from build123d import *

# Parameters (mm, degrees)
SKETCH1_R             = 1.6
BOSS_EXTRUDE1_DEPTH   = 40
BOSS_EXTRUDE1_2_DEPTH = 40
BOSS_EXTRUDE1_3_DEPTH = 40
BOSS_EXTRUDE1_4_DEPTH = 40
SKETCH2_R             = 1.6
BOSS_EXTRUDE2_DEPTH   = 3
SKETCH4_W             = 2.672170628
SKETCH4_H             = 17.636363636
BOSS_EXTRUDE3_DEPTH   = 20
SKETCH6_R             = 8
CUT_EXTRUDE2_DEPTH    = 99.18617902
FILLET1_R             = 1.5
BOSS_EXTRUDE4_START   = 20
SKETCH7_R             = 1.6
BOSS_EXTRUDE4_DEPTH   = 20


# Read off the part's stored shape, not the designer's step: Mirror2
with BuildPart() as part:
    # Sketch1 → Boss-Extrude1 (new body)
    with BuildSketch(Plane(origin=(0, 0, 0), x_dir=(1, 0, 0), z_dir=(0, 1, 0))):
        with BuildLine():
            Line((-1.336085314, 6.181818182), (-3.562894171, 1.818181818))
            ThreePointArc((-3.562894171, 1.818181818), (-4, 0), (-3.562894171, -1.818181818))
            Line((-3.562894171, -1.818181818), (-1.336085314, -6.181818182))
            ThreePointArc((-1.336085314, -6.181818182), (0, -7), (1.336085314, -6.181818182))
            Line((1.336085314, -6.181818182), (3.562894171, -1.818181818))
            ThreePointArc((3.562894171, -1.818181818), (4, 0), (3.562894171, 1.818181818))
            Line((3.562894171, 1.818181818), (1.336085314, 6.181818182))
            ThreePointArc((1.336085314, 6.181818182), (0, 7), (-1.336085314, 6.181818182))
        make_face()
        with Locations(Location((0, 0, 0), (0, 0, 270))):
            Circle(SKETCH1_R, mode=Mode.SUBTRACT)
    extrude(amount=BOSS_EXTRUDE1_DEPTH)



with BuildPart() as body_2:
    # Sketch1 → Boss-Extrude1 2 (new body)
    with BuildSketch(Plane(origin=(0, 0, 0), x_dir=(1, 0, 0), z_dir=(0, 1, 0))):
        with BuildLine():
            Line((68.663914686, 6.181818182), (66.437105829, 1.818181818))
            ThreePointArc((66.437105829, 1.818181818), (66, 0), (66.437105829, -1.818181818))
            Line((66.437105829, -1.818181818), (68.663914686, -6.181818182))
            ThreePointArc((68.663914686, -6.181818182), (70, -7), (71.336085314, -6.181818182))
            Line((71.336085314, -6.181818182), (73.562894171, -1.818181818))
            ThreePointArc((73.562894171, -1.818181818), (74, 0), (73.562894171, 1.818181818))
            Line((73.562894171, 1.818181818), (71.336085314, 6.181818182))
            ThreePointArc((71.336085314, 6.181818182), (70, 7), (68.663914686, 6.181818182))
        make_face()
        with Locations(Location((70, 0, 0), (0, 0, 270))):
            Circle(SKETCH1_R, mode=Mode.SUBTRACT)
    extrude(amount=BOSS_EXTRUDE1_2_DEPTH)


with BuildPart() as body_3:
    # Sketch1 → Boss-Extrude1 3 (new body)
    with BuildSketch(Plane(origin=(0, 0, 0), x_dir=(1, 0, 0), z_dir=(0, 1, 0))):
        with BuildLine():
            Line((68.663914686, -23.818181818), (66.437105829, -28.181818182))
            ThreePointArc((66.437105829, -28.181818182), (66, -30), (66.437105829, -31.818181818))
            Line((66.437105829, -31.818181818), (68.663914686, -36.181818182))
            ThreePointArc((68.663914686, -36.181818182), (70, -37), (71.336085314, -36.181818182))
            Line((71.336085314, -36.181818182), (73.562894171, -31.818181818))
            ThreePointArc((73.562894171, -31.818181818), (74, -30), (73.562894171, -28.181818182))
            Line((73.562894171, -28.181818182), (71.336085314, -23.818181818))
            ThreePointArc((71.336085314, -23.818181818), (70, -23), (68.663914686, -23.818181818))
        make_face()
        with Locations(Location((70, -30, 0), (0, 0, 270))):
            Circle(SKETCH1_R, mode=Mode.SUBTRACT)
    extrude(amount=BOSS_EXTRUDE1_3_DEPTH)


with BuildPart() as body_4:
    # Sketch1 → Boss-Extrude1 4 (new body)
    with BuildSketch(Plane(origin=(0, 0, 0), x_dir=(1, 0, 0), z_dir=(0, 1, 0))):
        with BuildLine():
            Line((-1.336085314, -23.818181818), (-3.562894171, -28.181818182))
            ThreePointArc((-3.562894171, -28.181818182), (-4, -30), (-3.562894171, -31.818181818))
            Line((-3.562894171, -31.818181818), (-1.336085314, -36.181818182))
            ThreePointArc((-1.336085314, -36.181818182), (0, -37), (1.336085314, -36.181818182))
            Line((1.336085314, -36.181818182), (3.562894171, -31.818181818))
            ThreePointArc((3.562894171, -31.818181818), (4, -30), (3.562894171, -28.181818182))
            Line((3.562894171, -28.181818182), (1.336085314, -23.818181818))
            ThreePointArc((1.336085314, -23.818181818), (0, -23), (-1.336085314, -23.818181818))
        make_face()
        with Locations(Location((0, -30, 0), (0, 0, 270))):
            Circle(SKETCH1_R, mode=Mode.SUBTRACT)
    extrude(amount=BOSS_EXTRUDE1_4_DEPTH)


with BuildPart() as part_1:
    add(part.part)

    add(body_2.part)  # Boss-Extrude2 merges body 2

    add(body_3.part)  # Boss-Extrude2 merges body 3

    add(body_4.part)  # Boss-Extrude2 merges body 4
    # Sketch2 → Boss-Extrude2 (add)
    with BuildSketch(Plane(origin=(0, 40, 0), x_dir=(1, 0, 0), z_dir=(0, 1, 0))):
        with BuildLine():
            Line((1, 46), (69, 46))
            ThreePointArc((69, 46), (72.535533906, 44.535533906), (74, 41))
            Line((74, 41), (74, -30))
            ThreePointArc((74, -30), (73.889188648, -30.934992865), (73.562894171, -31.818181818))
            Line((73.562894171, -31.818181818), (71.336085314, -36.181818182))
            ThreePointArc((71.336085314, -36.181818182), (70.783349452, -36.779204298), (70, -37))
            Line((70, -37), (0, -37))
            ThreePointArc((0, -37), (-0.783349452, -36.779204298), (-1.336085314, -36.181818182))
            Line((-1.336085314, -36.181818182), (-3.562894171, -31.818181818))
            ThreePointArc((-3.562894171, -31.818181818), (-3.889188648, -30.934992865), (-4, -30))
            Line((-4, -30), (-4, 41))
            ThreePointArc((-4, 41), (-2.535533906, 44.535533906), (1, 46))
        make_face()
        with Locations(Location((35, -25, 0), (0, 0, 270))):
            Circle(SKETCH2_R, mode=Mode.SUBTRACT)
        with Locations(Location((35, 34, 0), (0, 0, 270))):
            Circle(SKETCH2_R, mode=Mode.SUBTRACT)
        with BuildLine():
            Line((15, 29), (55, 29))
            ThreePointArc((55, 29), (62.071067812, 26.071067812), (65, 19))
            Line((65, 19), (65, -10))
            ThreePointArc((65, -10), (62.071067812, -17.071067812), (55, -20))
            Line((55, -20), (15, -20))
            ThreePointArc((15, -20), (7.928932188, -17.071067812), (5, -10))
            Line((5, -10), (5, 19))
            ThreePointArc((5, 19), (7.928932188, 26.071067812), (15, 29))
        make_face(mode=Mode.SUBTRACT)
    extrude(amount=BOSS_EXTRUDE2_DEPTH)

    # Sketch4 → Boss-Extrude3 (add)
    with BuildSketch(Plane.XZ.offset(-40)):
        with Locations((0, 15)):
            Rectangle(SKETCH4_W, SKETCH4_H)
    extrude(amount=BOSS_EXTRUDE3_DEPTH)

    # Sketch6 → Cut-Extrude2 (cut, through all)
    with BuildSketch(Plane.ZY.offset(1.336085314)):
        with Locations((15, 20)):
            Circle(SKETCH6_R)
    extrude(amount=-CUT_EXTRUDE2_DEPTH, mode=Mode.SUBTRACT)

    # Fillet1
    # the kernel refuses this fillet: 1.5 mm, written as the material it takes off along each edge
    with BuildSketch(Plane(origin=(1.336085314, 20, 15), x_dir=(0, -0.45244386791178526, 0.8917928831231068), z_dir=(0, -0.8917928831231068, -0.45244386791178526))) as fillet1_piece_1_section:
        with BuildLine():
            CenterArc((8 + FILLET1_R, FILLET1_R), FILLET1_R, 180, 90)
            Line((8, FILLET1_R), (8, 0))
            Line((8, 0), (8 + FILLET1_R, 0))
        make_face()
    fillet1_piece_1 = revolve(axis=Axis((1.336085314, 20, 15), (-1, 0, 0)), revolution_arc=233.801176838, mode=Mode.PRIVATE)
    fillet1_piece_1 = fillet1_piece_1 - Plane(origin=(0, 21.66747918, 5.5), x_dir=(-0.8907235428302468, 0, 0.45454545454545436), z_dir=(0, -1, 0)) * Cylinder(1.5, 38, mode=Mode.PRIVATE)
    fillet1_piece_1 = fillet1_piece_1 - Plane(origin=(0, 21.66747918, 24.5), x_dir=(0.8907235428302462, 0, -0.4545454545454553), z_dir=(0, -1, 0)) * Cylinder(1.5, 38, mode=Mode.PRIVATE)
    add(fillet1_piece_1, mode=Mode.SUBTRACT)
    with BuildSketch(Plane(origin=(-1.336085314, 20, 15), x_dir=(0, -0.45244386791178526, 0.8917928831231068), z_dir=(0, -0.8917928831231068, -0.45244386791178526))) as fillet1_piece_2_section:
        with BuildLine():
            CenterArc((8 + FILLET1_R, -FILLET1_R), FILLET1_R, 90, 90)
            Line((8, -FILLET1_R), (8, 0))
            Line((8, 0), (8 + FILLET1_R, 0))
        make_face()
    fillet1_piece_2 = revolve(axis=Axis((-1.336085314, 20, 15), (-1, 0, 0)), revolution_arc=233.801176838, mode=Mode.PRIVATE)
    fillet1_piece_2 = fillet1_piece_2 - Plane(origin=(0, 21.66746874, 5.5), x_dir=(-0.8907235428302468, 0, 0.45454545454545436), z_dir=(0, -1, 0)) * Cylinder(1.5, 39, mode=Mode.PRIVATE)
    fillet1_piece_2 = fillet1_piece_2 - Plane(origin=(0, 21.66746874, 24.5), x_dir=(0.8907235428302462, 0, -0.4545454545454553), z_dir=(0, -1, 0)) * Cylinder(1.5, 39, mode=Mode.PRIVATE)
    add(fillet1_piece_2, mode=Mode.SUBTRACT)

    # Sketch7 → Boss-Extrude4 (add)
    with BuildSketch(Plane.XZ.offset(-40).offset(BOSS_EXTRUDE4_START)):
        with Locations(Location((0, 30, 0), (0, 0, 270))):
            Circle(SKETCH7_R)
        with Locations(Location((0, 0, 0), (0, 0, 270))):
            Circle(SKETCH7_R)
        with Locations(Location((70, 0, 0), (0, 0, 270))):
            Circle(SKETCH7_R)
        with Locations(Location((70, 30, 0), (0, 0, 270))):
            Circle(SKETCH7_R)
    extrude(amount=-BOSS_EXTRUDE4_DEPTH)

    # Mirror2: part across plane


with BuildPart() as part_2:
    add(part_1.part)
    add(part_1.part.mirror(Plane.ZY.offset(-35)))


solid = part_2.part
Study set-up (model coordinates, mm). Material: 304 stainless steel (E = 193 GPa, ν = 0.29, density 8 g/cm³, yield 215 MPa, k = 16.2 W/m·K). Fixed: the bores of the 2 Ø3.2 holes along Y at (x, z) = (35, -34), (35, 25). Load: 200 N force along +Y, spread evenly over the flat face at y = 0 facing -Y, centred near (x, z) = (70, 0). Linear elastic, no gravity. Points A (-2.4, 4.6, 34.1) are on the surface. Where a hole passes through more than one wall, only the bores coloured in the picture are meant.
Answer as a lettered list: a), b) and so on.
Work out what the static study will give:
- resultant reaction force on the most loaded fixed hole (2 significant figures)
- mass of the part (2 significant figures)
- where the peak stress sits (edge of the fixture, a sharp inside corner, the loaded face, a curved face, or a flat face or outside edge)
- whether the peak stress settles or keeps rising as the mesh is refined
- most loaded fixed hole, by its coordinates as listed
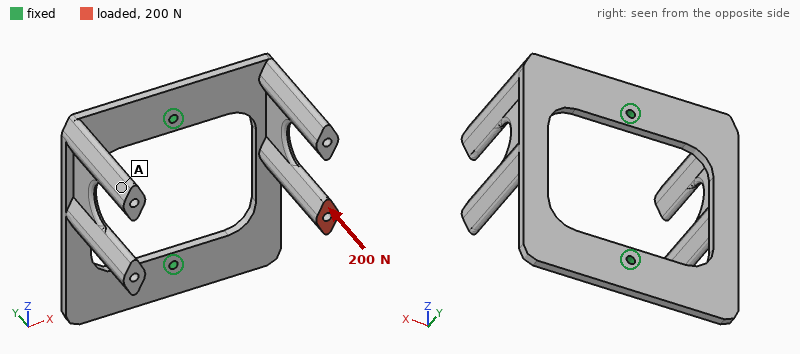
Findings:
a) 110 N
b) 180 g
c) edge of the fixture
d) keeps rising
e) (35, 25)
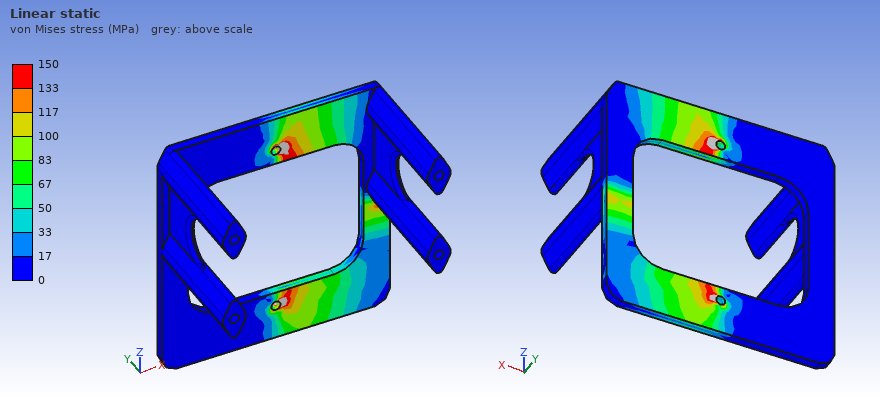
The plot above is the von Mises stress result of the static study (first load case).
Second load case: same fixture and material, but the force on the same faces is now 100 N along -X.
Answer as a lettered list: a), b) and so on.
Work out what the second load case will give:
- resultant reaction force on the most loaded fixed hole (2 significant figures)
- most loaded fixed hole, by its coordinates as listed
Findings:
a) 67 N
b) (35, 25)
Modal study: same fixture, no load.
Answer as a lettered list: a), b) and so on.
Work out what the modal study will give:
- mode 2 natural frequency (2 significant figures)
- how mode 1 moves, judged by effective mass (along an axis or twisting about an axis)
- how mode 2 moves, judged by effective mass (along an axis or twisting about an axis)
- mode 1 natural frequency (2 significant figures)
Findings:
a) 430 Hz
b) along X
c) along Y
d) 410 Hz
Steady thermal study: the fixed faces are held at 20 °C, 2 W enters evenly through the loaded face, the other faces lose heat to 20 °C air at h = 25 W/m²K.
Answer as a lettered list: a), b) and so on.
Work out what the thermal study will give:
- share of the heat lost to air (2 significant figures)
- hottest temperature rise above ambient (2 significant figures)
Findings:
a) 92 %
b) 54 K
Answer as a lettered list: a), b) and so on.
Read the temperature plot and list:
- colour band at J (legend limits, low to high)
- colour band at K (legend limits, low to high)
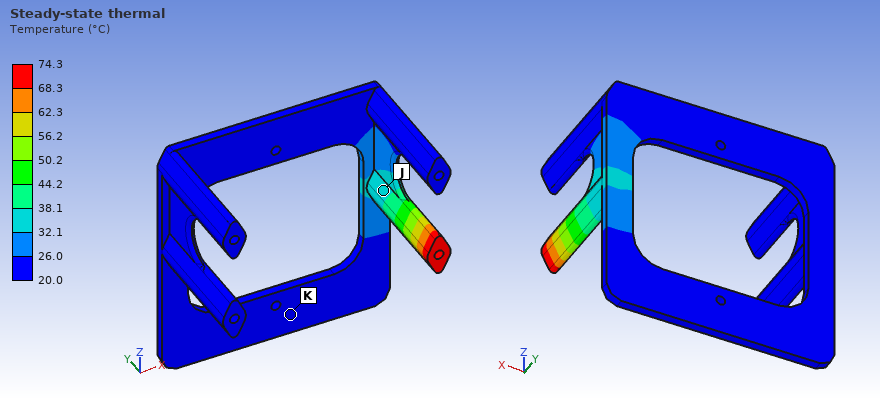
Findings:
a) 32.1 to 38.1 °C
b) 20.0 to 26.0 °C
